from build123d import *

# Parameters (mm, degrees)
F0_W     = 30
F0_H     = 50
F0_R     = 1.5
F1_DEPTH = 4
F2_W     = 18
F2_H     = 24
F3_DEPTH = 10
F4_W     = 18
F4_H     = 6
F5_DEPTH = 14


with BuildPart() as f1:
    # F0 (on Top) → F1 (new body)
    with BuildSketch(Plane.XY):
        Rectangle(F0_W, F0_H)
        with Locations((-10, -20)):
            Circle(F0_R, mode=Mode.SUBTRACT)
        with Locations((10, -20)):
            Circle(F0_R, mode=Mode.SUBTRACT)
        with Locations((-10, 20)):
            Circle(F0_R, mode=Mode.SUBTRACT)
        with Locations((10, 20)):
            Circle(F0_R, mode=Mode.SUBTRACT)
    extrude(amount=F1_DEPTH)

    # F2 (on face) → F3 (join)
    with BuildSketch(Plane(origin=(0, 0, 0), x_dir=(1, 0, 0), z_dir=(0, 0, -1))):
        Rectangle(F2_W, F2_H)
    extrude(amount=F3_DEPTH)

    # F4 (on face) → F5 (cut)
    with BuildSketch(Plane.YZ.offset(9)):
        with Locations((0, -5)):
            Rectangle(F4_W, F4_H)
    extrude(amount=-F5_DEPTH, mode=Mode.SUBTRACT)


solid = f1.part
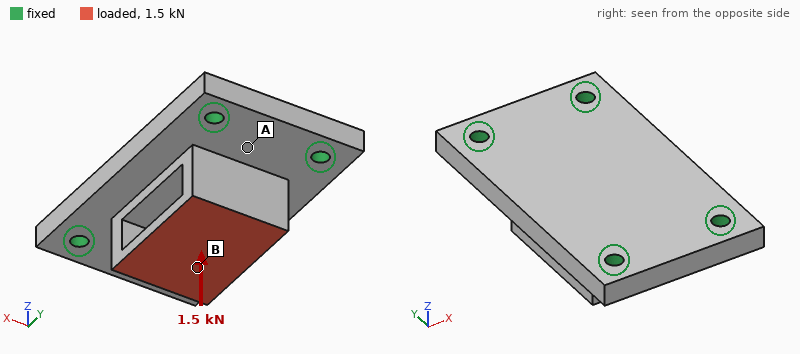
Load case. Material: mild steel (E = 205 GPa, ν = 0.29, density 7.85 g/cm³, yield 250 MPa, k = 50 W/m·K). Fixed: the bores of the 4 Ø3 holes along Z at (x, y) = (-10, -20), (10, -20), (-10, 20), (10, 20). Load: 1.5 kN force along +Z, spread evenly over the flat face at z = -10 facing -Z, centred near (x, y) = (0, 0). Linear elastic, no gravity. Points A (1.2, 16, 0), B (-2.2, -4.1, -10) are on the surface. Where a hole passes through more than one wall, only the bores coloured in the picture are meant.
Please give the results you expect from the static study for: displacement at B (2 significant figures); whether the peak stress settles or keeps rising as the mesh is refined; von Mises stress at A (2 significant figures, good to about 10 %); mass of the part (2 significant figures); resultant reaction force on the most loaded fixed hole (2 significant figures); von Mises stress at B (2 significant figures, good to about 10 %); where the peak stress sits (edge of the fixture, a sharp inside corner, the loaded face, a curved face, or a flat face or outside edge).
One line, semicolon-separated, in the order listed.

7.4 µm; keeps rising; 11 MPa; 68 g; 410 N; 39 MPa; edge of the fixture
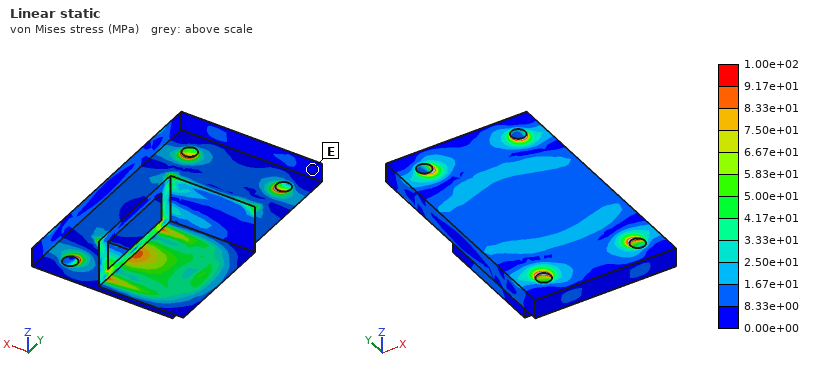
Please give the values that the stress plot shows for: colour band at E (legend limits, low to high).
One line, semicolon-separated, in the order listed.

0.00e+00 to 8.33e+00 MPa
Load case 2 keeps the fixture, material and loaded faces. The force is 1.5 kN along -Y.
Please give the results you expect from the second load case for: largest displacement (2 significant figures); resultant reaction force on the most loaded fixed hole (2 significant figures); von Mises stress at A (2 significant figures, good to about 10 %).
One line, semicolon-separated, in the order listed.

10 µm; 580 N; 14 MPa
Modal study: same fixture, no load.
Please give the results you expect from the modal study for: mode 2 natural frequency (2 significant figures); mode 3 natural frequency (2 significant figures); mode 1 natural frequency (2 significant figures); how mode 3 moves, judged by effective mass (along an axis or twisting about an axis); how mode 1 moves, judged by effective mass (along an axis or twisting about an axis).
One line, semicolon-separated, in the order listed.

14 kHz; 21 kHz; 12 kHz; along Y; along Z
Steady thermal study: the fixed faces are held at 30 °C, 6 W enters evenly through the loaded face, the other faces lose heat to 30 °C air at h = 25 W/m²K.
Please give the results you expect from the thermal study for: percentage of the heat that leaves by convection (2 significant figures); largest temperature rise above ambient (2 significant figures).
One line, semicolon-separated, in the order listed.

10.0 %; 17 K
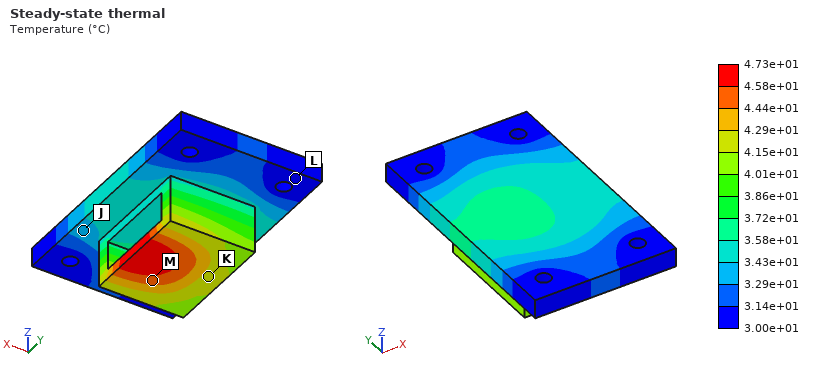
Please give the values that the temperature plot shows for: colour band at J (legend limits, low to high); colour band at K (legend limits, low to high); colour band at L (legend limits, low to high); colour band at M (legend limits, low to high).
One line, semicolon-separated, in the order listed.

3.29e+01 to 3.43e+01 °C; 4.15e+01 to 4.29e+01 °C; 3.00e+01 to 3.14e+01 °C; 4.44e+01 to 4.58e+01 °C
